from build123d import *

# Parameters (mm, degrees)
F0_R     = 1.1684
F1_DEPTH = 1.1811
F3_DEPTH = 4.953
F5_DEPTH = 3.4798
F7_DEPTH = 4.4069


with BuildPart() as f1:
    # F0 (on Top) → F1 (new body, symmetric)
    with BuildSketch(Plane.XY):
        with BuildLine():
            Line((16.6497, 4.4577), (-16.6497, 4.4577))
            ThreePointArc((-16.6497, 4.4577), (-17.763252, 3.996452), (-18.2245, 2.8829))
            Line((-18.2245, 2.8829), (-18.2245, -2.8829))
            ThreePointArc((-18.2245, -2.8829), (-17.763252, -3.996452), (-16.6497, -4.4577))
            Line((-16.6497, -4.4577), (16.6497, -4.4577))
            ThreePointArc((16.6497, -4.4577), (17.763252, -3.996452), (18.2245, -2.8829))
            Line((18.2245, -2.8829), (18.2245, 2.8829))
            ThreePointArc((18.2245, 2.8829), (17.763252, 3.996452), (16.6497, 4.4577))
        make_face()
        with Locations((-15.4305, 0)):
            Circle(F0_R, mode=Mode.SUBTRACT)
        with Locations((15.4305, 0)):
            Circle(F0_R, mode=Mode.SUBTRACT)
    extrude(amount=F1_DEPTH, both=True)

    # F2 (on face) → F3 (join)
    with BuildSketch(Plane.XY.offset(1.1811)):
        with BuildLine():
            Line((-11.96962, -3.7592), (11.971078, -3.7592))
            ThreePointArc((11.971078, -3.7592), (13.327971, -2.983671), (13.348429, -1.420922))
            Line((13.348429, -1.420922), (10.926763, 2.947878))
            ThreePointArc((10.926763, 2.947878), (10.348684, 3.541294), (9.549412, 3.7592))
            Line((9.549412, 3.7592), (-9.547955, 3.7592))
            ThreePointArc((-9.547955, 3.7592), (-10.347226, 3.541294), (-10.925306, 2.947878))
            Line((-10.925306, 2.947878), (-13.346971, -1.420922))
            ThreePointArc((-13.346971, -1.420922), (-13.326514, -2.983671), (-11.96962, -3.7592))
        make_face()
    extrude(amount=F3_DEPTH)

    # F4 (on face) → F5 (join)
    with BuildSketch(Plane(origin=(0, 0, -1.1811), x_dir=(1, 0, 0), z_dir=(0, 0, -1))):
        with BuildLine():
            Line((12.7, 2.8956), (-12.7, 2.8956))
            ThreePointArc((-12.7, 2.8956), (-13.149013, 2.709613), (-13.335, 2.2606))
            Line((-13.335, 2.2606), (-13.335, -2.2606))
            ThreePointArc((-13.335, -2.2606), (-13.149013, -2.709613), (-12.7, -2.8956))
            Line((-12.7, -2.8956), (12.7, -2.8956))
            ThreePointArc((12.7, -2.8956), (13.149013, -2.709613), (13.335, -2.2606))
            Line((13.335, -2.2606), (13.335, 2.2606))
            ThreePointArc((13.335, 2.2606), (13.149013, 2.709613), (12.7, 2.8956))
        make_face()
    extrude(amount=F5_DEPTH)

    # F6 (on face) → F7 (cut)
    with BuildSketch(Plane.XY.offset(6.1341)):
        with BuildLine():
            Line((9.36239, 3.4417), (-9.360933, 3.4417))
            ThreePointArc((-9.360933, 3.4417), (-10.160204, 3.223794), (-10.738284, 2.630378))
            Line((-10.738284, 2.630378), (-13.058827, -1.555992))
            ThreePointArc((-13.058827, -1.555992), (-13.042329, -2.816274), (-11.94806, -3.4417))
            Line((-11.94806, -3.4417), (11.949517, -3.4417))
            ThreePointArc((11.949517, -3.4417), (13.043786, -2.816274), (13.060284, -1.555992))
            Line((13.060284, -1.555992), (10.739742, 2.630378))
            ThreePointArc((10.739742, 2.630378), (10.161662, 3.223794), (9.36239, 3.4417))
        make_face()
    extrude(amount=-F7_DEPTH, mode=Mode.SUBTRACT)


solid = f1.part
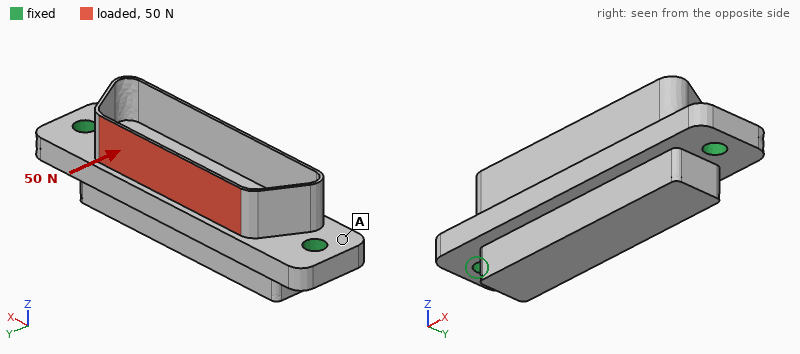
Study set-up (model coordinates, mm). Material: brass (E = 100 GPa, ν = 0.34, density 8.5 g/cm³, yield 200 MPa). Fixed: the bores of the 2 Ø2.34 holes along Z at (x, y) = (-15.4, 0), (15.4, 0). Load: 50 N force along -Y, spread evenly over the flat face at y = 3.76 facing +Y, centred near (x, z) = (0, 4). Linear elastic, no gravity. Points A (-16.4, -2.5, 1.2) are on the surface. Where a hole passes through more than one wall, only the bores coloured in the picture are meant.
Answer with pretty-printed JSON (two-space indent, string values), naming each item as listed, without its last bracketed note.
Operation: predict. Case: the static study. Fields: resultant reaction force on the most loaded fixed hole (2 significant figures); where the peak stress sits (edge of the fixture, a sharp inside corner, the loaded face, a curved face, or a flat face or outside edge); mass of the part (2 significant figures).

{
  "resultant reaction force on the most loaded fixed hole": "25 N",
  "where the peak stress sits": "the loaded face",
  "mass of the part": "12 g"
}
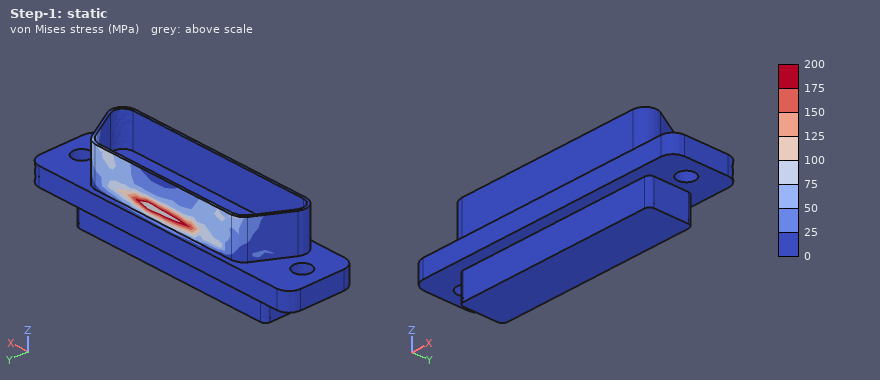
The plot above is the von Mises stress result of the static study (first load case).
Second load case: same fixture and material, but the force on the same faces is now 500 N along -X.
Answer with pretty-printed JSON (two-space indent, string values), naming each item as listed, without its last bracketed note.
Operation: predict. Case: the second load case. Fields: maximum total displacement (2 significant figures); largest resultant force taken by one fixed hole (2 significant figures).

{
  "maximum total displacement": "10 µm",
  "largest resultant force taken by one fixed hole": "270 N"
}
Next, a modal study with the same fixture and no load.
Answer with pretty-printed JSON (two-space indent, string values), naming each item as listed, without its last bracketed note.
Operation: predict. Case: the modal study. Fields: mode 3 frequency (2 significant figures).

{
  "mode 3 frequency": "13 kHz"
}
